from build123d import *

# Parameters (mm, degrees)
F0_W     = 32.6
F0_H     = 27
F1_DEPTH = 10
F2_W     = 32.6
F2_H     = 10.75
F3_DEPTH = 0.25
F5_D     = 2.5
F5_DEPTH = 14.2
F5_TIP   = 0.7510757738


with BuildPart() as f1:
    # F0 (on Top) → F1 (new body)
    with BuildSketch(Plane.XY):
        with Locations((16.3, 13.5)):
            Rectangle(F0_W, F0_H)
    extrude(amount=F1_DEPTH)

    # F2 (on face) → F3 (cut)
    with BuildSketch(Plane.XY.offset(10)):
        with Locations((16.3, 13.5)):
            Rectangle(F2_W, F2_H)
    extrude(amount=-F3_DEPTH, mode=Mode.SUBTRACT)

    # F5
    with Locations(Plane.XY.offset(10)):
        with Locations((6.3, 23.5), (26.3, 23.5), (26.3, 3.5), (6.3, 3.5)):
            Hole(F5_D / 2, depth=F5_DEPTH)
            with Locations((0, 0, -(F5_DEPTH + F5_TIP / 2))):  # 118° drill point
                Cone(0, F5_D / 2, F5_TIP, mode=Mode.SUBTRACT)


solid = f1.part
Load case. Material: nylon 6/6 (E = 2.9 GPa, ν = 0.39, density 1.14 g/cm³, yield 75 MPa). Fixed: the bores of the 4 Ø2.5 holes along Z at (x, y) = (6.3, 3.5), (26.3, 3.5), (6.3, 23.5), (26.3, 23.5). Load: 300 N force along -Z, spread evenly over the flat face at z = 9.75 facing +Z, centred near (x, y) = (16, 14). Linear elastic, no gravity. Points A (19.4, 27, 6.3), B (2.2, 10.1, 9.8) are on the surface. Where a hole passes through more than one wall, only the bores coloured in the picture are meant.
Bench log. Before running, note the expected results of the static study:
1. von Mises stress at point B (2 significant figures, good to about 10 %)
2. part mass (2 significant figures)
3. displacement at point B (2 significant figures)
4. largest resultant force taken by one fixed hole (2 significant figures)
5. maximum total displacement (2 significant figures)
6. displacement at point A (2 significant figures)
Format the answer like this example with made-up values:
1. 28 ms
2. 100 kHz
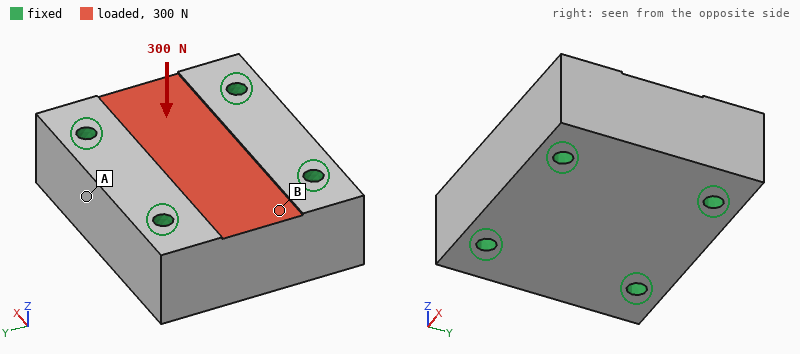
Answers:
1. 0.97 MPa
2. 9.7 g
3. 6.5 µm
4. 76 N
5. 8.1 µm
6. 1.3 µm
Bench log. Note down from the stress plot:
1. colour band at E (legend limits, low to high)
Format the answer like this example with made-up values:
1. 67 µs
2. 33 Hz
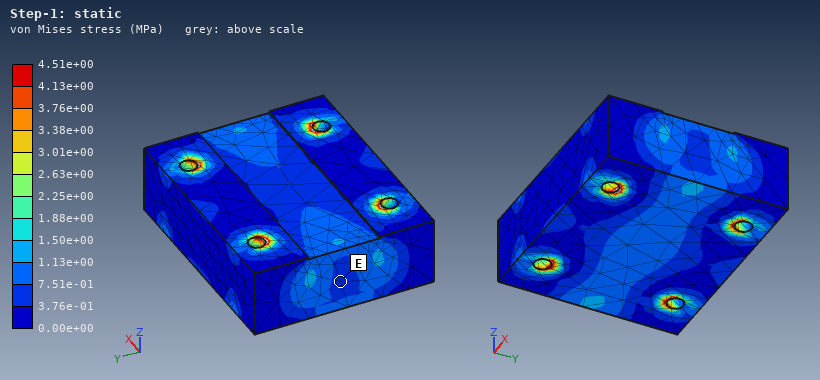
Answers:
1. 3.76e-01 to 7.51e-01 MPa
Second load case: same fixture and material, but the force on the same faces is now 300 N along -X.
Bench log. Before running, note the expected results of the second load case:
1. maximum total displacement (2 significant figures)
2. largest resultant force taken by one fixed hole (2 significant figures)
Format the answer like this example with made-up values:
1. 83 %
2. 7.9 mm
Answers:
1. 12 µm
2. 80 N
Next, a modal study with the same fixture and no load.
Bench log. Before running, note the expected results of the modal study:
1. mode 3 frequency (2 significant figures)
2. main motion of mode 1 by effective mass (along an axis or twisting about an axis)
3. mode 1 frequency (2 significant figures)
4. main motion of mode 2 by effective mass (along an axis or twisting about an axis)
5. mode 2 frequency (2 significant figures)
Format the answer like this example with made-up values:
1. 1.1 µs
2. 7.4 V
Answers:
1. 20 kHz
2. along Z
3. 15 kHz
4. twisting about Y
5. 18 kHz
